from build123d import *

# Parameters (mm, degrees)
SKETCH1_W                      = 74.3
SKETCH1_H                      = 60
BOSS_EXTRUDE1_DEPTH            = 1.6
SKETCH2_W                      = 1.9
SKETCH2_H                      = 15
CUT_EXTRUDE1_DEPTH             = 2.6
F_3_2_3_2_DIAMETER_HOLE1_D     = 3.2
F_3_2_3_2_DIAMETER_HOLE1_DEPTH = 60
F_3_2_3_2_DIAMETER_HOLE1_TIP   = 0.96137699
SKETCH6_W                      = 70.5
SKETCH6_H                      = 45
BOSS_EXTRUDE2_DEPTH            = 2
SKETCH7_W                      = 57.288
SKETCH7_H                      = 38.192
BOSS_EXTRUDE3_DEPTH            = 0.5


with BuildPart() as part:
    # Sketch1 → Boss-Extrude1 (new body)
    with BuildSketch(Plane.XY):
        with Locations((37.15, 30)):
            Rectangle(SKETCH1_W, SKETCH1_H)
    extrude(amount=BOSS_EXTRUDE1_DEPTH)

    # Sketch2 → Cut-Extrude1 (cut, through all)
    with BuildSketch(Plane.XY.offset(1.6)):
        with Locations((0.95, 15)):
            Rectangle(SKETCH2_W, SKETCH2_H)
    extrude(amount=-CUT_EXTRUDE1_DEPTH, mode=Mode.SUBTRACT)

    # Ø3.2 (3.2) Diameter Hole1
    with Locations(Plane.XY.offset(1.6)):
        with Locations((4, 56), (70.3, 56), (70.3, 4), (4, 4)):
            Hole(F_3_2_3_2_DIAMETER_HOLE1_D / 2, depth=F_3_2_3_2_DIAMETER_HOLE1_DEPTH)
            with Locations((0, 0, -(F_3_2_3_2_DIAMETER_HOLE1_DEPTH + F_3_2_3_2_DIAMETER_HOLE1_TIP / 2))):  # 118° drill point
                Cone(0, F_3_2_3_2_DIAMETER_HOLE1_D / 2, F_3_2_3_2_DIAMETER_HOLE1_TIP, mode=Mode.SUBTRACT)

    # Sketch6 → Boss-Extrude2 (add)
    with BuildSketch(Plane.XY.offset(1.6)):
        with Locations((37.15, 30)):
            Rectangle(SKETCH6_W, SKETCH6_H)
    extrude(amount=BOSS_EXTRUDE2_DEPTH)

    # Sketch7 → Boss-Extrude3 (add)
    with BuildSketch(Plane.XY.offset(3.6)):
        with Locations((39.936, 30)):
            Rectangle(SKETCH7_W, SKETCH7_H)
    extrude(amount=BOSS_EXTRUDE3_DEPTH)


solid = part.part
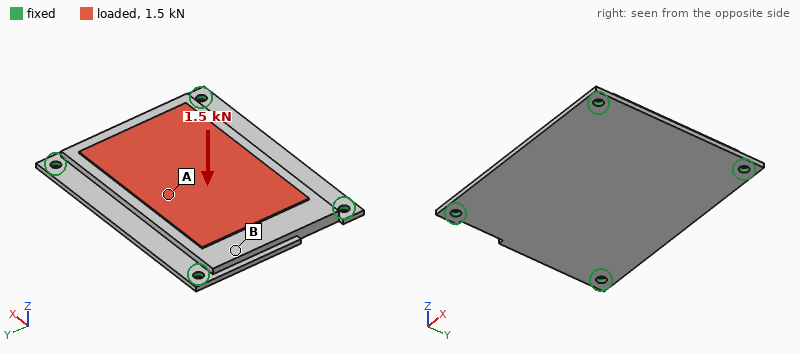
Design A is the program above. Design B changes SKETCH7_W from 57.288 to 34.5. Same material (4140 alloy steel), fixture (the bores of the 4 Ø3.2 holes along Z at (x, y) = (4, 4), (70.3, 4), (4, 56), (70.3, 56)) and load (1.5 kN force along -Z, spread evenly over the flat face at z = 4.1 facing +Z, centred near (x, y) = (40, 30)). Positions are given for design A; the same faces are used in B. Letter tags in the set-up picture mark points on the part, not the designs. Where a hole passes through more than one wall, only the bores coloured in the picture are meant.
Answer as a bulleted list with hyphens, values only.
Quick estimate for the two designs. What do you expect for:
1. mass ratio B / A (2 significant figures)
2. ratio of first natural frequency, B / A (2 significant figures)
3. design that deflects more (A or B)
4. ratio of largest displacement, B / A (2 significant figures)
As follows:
- 0.97
- 0.98
- B
- 1.3
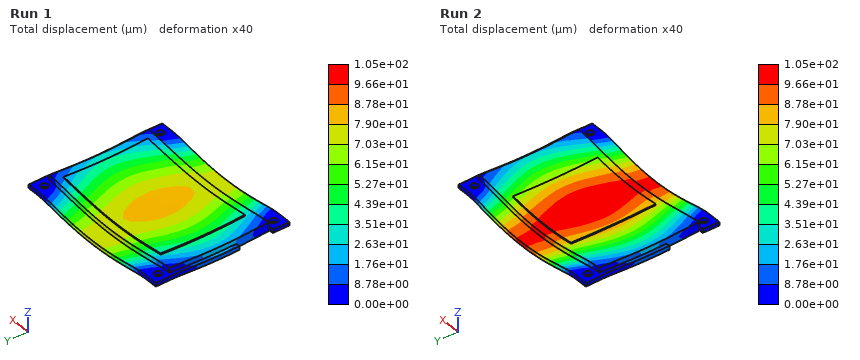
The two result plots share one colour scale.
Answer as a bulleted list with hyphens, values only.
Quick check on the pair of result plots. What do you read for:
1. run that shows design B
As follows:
- Run 2
